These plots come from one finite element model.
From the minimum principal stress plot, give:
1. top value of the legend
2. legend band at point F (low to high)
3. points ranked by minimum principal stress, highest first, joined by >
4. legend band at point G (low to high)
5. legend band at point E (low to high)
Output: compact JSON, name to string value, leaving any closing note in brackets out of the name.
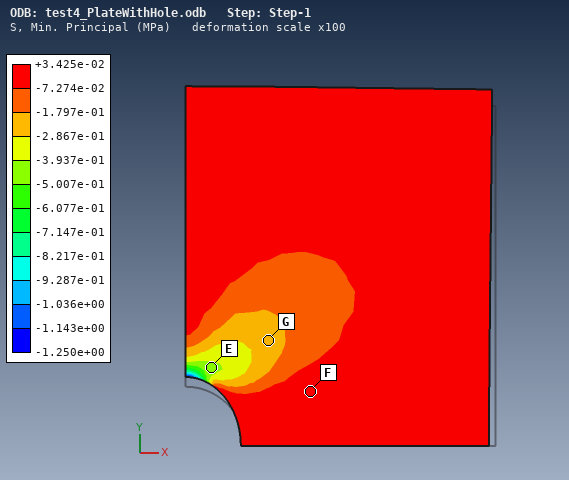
{"top value of the legend": "+3.425e-02 MPa", "legend band at point F": "-7.274e-02 to +3.425e-02 MPa", "points ranked by minimum principal stress, highest first, joined by >": "F > G > E", "legend band at point G": "-2.867e-01 to -1.797e-01 MPa", "legend band at point E": "-5.007e-01 to -3.937e-01 MPa"}
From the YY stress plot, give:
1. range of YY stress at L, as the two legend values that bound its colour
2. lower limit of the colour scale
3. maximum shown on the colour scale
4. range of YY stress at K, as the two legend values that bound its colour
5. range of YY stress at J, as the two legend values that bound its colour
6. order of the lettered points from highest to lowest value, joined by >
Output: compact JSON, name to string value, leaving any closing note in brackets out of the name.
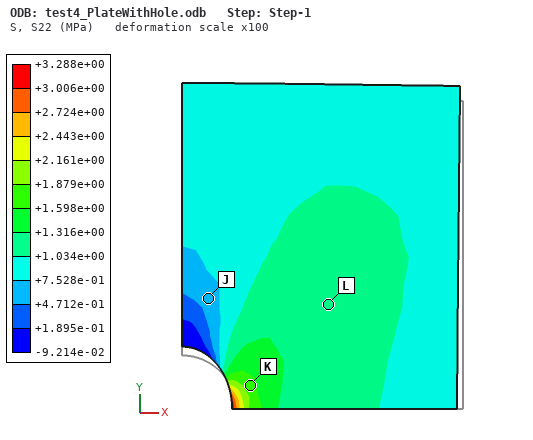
{"range of YY stress at L, as the two legend values that bound its colour": "+1.034e+00 to +1.316e+00 MPa", "lower limit of the colour scale": "-9.214e-02 MPa", "maximum shown on the colour scale": "+3.288e+00 MPa", "range of YY stress at K, as the two legend values that bound its colour": "+1.598e+00 to +1.879e+00 MPa", "range of YY stress at J, as the two legend values that bound its colour": "+4.712e-01 to +7.528e-01 MPa", "order of the lettered points from highest to lowest value, joined by >": "K > L > J"}
